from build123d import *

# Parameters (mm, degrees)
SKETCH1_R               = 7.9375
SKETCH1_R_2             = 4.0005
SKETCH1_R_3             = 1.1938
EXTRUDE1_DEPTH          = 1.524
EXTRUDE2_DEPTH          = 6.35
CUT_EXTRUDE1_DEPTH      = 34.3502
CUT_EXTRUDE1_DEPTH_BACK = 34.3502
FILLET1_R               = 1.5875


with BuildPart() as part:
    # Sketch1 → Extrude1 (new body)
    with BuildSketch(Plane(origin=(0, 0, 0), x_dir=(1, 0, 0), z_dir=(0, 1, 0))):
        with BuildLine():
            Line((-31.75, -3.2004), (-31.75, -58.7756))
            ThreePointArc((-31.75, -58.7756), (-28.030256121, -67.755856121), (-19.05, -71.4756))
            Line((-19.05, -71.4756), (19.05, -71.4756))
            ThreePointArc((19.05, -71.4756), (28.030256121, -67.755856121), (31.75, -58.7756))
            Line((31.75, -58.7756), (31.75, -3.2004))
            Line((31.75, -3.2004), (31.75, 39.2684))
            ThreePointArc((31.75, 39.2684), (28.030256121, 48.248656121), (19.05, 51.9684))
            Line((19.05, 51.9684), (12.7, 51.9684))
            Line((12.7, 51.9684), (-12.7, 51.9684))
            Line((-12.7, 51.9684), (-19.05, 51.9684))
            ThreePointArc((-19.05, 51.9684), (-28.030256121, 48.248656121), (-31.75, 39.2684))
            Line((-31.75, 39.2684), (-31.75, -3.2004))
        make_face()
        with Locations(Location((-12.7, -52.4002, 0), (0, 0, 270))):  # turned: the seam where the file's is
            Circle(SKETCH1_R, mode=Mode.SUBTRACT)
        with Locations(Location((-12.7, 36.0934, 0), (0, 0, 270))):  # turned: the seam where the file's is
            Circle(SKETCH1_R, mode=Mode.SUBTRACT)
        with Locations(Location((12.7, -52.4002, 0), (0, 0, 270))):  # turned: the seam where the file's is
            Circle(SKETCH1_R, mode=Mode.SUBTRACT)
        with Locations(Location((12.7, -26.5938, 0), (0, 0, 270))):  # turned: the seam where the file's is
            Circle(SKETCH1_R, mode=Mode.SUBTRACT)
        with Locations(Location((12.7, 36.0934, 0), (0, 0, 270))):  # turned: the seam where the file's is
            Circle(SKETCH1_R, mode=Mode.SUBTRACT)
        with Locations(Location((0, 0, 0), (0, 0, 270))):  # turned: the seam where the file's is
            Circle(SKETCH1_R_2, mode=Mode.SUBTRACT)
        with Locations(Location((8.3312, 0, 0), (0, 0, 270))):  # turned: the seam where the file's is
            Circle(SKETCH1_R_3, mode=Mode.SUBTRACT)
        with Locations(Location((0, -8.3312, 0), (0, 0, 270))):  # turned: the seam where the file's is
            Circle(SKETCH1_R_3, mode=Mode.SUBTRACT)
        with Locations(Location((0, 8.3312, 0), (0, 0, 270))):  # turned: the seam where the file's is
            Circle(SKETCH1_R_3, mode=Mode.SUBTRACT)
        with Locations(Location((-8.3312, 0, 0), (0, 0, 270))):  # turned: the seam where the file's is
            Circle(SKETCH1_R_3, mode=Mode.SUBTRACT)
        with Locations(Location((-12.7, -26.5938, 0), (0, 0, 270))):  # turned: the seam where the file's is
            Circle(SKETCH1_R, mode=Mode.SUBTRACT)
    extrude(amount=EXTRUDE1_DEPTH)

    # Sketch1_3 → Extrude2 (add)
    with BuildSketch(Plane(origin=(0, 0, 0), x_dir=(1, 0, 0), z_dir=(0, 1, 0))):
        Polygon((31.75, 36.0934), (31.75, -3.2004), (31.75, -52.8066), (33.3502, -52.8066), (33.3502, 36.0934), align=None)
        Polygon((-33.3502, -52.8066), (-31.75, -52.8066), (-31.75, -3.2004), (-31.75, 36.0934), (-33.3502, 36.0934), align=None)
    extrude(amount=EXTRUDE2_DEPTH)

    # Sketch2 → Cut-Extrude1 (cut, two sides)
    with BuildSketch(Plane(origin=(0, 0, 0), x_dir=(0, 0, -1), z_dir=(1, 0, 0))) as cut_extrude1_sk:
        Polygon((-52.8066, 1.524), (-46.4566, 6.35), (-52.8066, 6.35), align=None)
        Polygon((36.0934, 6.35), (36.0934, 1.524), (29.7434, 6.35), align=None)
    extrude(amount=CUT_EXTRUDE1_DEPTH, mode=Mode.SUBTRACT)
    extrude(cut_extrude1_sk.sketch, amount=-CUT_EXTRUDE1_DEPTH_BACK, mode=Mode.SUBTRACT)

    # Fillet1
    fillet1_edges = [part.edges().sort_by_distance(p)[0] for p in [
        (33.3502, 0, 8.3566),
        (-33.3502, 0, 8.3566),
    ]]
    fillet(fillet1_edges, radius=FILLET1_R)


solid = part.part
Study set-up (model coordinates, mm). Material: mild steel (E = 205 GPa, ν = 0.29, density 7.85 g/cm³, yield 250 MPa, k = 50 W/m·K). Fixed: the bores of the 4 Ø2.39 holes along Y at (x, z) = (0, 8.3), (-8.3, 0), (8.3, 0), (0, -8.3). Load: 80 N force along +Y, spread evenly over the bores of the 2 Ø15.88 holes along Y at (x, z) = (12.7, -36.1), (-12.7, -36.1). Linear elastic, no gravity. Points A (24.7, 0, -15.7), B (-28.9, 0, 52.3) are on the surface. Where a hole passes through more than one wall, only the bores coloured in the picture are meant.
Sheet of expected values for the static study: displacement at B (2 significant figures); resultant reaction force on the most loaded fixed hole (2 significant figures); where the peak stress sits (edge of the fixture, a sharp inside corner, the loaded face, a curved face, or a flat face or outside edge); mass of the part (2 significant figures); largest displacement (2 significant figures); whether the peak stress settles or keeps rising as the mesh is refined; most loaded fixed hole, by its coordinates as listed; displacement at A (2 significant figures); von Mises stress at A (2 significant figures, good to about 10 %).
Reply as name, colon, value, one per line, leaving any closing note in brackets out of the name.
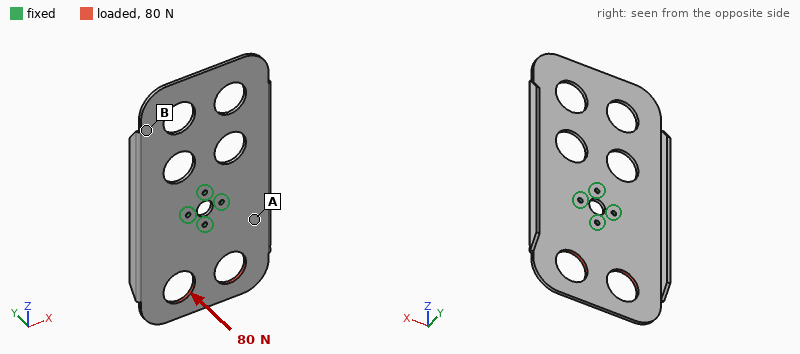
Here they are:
displacement at B: 0.13 mm
resultant reaction force on the most loaded fixed hole: 120 N
where the peak stress sits: edge of the fixture
mass of the part: 90 g
largest displacement: 0.27 mm
whether the peak stress settles or keeps rising as the mesh is refined: keeps rising
most loaded fixed hole, by its coordinates as listed: (0, -8.3)
displacement at A: 0.060 mm
von Mises stress at A: 20 MPa
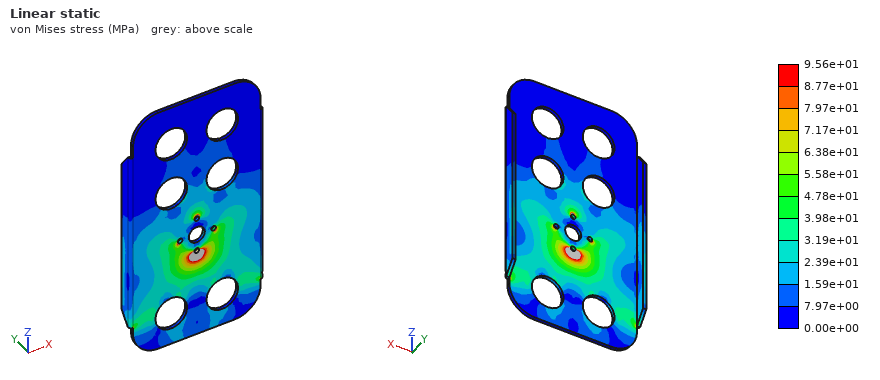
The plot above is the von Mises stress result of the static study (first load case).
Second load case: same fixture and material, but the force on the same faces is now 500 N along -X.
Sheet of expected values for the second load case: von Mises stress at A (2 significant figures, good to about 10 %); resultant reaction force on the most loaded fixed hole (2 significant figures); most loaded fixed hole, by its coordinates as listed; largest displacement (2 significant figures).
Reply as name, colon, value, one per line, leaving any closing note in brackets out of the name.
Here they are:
von Mises stress at A: 6.4 MPa
resultant reaction force on the most loaded fixed hole: 710 N
most loaded fixed hole, by its coordinates as listed: (0, -8.3)
largest displacement: 15 µm
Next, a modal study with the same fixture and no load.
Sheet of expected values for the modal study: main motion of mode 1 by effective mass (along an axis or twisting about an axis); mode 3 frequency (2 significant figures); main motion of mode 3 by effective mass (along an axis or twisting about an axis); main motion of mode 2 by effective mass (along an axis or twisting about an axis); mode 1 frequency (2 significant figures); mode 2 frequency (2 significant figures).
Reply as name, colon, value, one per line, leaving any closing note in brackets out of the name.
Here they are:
main motion of mode 1 by effective mass: along Y
mode 3 frequency: 830 Hz
main motion of mode 3 by effective mass: along Y
main motion of mode 2 by effective mass: twisting about Z
mode 1 frequency: 380 Hz
mode 2 frequency: 600 Hz
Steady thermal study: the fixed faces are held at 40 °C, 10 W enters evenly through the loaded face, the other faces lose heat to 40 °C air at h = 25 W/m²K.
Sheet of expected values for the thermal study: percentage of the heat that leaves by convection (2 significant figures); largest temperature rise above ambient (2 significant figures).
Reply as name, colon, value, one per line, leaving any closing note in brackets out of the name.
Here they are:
percentage of the heat that leaves by convection: 53 %
largest temperature rise above ambient: 59 K
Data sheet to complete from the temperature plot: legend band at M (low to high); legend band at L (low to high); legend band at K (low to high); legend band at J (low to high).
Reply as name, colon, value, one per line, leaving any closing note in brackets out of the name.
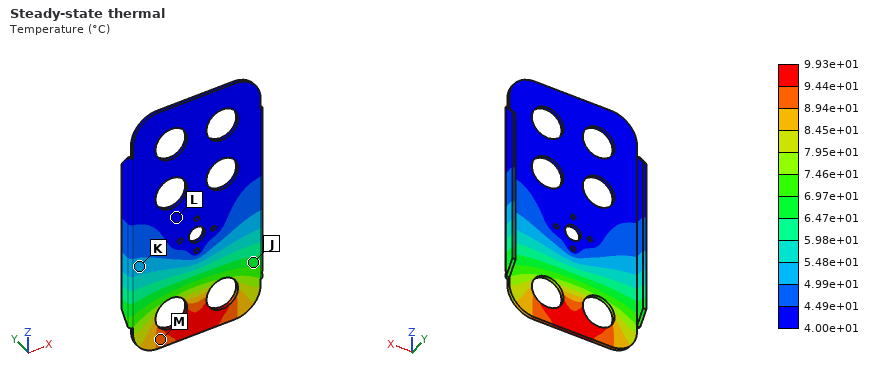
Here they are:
legend band at M: 8.94e+01 to 9.44e+01 °C
legend band at L: 4.00e+01 to 4.49e+01 °C
legend band at K: 4.99e+01 to 5.48e+01 °C
legend band at J: 6.47e+01 to 6.97e+01 °C
